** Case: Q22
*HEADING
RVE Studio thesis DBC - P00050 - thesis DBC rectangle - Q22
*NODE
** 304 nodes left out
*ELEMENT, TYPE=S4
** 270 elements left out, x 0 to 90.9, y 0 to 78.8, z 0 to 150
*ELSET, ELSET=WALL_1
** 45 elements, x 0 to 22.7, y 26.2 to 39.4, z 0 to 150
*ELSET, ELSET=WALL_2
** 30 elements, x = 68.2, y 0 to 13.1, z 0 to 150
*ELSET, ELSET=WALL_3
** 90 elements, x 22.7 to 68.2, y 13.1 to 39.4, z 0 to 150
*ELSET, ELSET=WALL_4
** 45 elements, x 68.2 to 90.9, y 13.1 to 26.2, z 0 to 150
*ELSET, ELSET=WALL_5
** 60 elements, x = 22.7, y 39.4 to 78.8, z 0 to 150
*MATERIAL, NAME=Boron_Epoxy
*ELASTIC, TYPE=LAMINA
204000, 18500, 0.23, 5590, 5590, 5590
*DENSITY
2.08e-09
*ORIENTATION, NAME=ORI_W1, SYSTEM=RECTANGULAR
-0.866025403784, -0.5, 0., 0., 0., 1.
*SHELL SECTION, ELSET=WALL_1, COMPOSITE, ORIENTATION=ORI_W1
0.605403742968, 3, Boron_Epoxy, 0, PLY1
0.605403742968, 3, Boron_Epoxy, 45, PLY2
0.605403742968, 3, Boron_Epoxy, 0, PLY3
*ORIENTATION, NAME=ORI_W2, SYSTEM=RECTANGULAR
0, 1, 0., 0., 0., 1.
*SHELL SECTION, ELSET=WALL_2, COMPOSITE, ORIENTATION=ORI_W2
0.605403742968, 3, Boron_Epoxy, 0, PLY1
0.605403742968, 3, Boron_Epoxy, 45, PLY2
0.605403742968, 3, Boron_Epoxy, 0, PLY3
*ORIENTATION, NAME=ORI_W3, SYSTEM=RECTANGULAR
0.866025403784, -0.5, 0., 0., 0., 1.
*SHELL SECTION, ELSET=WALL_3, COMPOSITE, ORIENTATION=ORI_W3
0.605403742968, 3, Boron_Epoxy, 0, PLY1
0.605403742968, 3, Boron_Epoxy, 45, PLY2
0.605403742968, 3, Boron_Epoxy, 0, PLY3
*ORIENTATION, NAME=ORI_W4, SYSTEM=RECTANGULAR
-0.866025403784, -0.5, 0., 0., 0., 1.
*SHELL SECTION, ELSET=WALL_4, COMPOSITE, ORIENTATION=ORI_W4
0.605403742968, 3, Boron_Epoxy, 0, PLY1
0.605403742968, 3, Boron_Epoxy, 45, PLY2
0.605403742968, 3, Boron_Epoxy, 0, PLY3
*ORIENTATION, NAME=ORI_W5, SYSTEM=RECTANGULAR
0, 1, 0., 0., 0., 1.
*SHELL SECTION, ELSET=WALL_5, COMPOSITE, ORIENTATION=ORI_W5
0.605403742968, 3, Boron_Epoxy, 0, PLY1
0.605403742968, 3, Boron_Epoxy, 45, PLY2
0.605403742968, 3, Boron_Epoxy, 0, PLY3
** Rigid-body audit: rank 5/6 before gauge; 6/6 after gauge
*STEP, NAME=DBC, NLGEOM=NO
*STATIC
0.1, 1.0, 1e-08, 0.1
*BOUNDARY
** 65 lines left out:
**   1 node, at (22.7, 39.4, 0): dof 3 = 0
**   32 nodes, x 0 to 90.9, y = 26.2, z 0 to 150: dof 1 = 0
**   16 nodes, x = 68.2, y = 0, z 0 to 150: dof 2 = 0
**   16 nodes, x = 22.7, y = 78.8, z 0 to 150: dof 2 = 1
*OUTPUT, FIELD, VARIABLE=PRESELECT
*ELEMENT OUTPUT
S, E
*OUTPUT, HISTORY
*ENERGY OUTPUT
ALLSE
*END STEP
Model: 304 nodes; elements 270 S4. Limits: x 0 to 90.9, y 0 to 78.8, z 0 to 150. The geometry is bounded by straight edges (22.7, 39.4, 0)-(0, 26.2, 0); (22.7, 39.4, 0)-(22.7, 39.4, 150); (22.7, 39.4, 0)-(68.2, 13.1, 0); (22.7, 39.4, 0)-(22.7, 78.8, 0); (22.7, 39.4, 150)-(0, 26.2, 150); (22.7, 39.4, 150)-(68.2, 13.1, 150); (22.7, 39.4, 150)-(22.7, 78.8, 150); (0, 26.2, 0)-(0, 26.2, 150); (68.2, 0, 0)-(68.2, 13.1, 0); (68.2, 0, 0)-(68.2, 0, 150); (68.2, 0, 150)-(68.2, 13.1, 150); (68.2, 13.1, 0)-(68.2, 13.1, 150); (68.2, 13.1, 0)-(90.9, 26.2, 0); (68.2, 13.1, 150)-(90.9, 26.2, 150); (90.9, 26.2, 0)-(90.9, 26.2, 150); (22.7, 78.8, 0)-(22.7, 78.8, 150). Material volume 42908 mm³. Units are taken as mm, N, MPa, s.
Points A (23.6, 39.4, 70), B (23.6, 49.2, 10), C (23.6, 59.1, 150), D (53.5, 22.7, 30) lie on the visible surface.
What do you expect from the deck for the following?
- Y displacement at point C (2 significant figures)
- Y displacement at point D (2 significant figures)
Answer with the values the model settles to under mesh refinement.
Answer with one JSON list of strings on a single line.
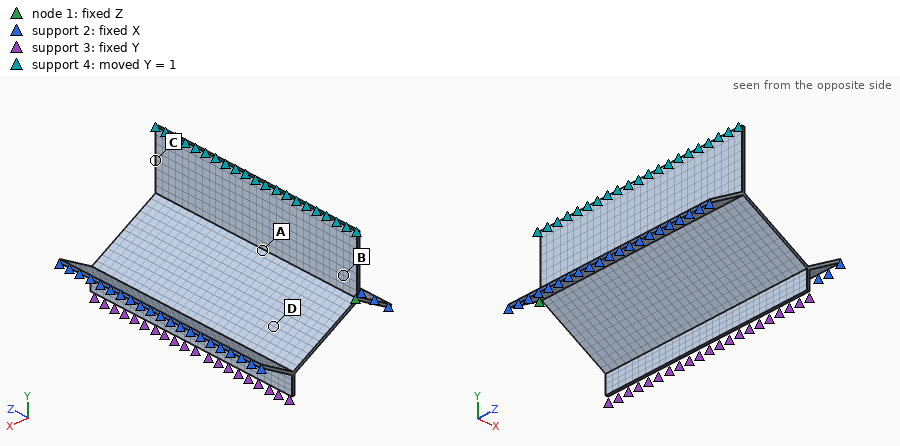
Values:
["0.98 mm", "0.32 mm"]
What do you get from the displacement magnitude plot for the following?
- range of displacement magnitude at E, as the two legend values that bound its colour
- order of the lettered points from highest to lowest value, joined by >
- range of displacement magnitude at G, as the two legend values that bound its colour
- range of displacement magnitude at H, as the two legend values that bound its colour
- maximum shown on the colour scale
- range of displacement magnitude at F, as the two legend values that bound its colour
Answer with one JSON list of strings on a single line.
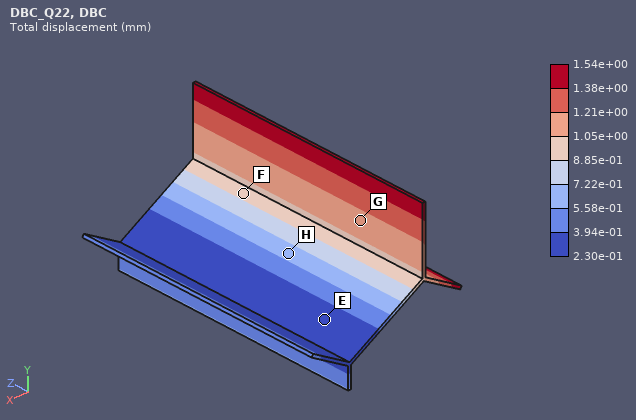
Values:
["2.30e-01 to 3.94e-01 mm", "G > F > H > E", "1.05e+00 to 1.21e+00 mm", "5.58e-01 to 7.22e-01 mm", "1.54e+00 mm", "8.85e-01 to 1.05e+00 mm"]
